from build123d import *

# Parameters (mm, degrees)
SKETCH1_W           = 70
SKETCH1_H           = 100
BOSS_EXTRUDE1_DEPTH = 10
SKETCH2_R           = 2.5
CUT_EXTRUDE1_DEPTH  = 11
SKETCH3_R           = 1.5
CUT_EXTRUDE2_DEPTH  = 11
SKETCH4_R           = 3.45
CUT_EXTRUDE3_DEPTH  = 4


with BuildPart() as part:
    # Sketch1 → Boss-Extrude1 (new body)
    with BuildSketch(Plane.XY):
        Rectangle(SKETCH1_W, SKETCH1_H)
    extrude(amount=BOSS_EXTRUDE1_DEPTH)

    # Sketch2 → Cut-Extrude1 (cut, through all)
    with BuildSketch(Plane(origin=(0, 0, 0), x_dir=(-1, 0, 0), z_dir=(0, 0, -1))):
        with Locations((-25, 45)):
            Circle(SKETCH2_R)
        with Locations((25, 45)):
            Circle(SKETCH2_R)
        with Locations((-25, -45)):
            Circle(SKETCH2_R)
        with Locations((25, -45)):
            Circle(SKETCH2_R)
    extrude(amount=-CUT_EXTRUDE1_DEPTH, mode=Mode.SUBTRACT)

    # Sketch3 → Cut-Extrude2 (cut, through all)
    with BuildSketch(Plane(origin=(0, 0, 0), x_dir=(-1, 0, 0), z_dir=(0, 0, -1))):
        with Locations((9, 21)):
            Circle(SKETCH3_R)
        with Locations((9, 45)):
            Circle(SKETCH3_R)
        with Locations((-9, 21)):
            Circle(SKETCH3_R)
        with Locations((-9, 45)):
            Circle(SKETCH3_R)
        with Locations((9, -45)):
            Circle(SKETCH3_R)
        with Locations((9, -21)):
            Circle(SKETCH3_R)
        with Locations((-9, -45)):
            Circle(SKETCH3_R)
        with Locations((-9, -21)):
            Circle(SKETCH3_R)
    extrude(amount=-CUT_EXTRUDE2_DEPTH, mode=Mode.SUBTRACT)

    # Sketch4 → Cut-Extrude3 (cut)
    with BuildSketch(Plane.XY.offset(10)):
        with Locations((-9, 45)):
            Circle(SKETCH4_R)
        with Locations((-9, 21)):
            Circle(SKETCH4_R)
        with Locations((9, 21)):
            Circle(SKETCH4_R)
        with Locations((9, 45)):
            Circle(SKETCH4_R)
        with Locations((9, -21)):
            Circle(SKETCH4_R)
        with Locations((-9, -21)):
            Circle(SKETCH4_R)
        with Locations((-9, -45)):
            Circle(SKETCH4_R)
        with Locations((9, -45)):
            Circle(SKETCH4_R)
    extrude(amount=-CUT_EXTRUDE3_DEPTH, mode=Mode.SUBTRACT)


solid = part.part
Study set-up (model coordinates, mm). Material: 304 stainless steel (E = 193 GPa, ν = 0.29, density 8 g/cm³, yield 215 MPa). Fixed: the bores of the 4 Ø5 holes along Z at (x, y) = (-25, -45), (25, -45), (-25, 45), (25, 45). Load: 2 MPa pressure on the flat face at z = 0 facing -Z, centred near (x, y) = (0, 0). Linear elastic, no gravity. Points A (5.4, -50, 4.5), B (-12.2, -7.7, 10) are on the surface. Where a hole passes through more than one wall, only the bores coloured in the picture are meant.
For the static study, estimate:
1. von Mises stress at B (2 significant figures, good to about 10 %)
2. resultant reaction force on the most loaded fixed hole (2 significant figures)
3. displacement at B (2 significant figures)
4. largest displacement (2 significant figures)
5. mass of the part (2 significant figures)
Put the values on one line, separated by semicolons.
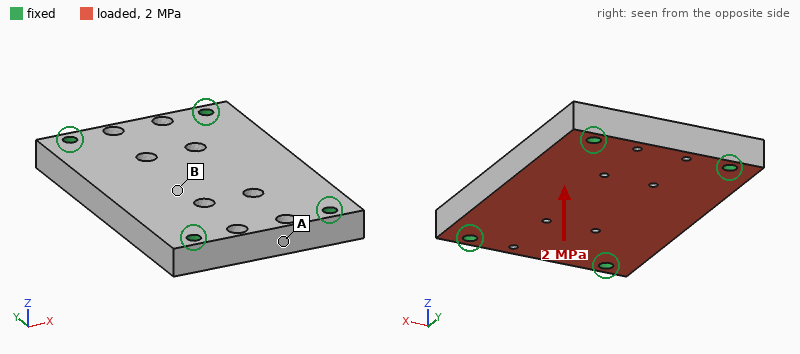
39 MPa; 3.4 kN; 33 µm; 34 µm; 540 g
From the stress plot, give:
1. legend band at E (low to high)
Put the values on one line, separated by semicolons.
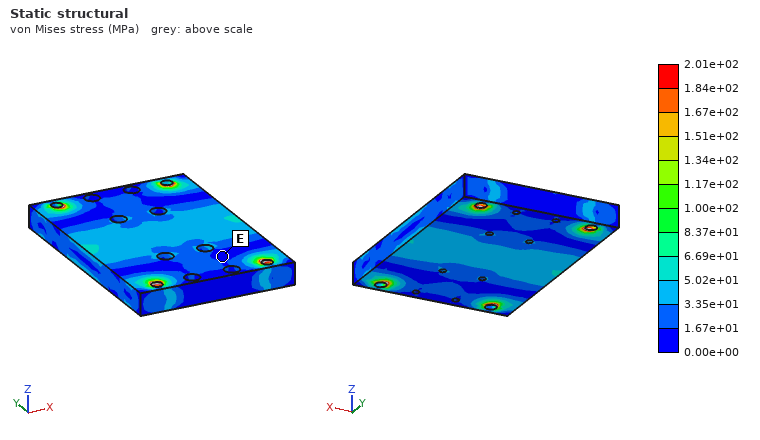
0.00e+00 to 1.67e+01 MPa
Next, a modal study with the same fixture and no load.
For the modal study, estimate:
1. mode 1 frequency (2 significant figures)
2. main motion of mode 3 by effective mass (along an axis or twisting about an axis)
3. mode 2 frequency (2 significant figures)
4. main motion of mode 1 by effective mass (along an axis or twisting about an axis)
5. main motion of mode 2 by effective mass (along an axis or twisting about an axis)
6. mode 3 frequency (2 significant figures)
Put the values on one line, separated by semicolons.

4900 Hz; twisting about X; 7100 Hz; along Z; twisting about Y; 12 kHz
